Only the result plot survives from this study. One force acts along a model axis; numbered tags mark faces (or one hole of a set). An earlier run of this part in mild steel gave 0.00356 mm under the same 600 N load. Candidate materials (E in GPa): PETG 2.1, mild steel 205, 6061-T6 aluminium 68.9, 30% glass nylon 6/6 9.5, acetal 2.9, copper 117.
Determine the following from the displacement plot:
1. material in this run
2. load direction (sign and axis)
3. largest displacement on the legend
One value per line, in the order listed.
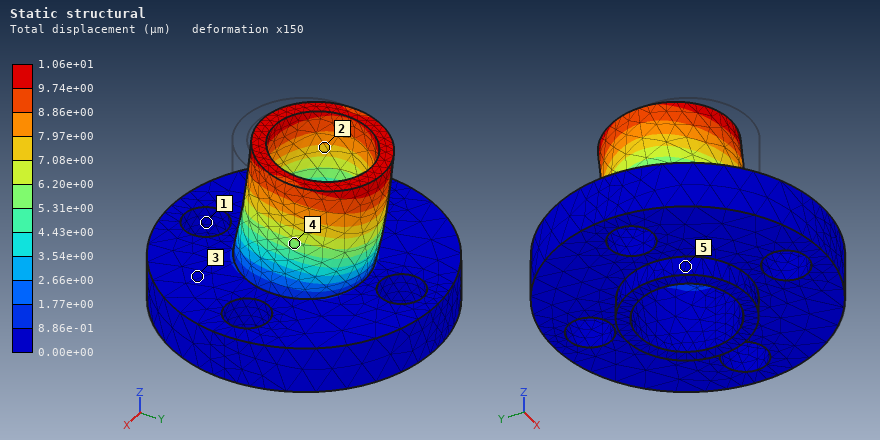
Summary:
6061-T6 aluminium
+Y
1.06e+01 µm
